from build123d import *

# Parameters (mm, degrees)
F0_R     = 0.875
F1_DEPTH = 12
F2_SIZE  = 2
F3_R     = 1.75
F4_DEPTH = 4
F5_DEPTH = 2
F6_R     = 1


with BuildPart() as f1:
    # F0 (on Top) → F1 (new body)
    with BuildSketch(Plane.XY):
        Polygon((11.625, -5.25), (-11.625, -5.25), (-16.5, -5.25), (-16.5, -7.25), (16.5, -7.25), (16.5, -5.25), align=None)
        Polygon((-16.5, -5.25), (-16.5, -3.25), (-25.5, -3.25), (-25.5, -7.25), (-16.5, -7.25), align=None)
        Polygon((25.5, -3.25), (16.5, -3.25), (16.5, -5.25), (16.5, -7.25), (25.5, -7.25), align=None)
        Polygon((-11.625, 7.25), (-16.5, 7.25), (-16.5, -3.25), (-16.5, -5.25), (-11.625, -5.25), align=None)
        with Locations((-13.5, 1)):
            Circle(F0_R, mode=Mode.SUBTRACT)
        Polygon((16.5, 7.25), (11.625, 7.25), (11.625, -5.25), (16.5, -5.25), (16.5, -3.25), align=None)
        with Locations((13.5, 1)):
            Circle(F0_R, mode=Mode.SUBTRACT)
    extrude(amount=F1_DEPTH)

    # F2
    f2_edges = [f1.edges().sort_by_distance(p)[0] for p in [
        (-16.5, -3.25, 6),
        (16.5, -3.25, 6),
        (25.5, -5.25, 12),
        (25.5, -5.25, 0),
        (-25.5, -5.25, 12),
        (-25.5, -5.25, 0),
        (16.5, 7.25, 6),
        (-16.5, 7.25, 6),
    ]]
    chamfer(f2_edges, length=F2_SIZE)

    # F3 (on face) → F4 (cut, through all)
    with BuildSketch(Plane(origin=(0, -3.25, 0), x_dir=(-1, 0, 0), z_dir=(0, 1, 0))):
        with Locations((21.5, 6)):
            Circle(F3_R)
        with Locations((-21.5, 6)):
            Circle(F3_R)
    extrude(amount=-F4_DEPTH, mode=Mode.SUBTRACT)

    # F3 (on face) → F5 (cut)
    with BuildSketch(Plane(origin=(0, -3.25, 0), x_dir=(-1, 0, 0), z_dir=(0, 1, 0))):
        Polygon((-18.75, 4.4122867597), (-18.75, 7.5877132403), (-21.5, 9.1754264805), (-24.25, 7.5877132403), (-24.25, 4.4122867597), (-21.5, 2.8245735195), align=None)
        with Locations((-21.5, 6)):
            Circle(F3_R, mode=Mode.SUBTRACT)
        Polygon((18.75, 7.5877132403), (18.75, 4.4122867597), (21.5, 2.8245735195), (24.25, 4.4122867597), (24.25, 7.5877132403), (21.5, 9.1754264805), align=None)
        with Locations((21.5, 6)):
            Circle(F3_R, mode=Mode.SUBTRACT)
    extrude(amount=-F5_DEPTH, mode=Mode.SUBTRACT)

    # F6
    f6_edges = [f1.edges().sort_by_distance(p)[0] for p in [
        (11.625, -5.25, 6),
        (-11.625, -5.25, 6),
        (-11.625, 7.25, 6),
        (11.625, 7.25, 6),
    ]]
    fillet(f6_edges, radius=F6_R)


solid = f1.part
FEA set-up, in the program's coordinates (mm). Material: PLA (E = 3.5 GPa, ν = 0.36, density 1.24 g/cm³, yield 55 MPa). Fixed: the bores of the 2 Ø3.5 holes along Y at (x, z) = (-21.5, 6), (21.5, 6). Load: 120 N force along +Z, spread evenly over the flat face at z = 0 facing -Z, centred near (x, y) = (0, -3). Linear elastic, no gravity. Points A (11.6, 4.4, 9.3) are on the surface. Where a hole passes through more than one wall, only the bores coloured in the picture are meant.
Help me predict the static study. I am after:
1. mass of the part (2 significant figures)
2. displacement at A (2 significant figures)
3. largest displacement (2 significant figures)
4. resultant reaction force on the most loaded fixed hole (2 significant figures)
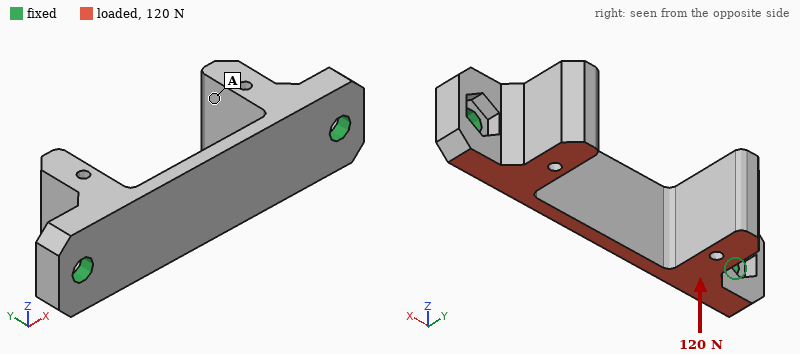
3.6 g
0.090 mm
0.11 mm
60 N
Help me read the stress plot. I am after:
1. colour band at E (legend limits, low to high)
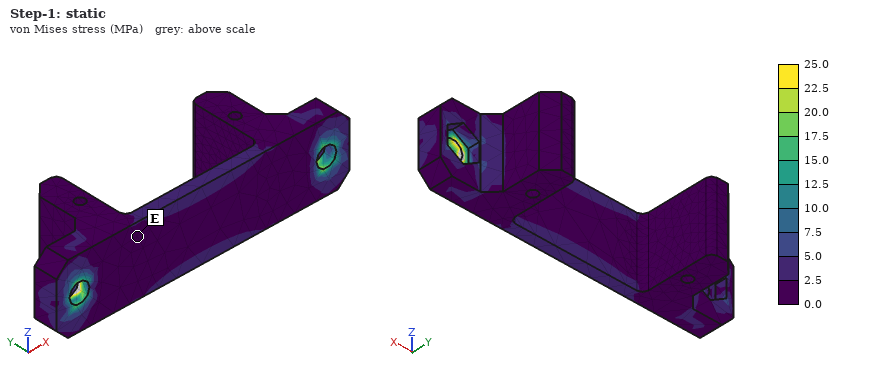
0.0 to 2.5 MPa
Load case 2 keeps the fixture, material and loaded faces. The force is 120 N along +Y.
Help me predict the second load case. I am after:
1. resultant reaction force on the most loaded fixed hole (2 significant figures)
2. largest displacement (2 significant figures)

61 N
0.35 mm
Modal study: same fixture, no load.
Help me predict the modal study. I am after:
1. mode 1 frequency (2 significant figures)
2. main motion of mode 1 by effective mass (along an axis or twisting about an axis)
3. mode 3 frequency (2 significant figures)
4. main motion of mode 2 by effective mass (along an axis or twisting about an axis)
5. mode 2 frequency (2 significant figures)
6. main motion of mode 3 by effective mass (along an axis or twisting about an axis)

2100 Hz
along Y
3300 Hz
along X
3100 Hz
along Z
